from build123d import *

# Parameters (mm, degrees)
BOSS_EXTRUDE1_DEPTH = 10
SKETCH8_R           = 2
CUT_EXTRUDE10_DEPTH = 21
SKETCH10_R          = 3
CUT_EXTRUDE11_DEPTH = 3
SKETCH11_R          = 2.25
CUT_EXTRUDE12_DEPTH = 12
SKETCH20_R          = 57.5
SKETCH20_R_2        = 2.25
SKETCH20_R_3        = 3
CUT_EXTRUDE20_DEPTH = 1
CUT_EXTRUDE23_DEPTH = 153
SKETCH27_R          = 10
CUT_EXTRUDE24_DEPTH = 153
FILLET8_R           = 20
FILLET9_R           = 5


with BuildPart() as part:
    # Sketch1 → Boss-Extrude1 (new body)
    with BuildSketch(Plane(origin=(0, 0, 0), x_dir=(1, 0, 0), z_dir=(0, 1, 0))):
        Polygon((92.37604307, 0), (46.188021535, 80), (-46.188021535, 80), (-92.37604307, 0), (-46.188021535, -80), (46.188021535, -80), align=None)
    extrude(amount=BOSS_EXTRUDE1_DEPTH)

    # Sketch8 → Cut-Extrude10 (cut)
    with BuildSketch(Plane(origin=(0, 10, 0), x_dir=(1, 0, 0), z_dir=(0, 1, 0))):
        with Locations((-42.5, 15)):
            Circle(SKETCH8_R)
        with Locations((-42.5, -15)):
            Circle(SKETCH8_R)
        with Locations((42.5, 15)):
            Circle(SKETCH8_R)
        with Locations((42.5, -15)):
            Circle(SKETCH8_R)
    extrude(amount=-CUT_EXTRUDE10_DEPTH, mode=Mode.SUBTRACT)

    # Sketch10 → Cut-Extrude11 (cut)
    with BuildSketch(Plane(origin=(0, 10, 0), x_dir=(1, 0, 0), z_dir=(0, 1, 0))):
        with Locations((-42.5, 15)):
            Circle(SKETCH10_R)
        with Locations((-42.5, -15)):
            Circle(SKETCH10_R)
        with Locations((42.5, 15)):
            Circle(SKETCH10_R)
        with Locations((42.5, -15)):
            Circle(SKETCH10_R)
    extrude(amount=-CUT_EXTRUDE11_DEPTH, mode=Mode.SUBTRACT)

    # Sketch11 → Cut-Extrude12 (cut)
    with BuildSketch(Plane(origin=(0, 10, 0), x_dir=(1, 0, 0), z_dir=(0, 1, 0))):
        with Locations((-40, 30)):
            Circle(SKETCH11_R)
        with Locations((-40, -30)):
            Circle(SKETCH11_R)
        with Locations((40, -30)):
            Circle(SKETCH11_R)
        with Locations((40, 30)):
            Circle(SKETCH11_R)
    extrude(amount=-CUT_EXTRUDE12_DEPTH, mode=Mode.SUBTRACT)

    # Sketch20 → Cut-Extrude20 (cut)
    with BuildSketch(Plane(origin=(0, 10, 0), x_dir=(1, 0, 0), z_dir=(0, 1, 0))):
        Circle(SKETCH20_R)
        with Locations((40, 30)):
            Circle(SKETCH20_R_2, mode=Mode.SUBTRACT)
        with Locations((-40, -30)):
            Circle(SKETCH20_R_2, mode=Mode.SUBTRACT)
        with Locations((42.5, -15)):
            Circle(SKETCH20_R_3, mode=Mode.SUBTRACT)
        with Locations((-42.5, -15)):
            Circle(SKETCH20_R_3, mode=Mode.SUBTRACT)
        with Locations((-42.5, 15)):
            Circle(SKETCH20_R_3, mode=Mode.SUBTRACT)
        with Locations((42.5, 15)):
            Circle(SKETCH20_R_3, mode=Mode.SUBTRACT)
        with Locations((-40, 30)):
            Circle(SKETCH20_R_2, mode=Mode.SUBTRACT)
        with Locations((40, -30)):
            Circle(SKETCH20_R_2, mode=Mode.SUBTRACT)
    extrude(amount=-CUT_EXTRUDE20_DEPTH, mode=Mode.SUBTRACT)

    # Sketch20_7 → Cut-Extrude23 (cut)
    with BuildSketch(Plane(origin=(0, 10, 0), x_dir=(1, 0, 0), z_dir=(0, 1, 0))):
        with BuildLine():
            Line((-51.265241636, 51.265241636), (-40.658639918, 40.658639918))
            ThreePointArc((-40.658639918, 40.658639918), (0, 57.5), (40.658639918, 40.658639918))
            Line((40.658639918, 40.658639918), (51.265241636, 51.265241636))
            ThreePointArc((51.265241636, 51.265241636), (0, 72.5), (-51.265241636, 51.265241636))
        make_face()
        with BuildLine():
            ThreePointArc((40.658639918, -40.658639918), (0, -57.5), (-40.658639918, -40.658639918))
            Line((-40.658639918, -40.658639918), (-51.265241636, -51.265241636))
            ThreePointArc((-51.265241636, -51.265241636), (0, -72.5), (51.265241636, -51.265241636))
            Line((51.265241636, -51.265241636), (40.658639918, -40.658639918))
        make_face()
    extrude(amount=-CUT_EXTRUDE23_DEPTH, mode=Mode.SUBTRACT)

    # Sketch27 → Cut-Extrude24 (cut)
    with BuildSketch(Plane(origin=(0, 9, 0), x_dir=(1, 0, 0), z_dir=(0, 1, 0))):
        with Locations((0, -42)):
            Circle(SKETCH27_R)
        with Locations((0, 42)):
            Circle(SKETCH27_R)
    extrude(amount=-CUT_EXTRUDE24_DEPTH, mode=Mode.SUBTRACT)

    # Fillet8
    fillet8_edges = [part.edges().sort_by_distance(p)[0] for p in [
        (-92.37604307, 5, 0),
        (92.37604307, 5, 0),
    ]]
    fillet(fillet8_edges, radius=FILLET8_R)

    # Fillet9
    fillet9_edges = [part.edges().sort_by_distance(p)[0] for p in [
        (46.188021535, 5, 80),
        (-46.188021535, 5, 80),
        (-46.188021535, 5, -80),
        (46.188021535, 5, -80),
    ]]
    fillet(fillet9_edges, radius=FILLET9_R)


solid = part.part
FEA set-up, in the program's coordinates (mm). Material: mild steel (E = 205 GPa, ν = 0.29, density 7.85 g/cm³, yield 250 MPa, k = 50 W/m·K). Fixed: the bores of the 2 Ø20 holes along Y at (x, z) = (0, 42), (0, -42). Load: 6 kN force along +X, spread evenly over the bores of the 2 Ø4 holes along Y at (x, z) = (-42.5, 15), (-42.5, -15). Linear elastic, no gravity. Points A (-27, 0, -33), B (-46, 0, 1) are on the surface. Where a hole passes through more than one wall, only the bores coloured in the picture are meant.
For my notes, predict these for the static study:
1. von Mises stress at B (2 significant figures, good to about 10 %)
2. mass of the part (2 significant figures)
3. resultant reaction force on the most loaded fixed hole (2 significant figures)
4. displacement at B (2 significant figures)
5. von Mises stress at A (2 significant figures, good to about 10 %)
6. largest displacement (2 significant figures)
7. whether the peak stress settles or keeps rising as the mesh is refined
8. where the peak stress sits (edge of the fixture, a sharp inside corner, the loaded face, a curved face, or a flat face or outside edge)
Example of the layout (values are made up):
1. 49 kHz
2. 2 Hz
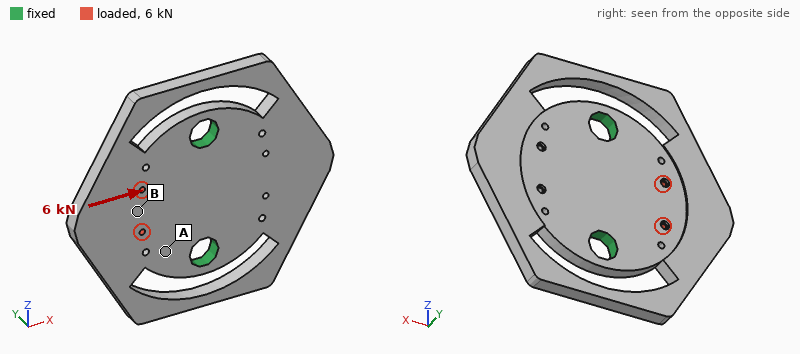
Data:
1. 4.1 MPa
2. 1.4 kg
3. 3.1 kN
4. 4.6 µm
5. 11 MPa
6. 11 µm
7. keeps rising
8. a sharp inside corner
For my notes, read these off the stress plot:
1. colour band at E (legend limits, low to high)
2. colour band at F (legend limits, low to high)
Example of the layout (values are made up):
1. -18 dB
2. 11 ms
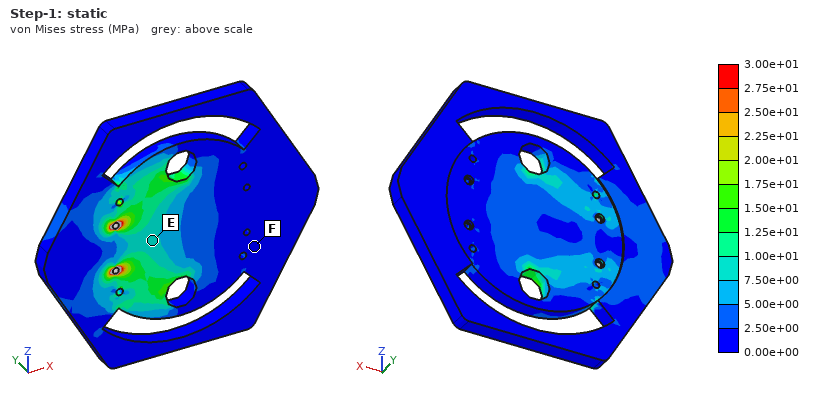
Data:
1. 7.50e+00 to 1.00e+01 MPa
2. 0.00e+00 to 2.50e+00 MPa
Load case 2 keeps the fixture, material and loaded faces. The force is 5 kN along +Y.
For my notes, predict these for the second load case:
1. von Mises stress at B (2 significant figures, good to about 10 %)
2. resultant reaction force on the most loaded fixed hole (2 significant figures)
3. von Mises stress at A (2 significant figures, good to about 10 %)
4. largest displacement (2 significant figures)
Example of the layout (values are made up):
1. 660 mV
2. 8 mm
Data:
1. 22 MPa
2. 2.5 kN
3. 58 MPa
4. 0.21 mm
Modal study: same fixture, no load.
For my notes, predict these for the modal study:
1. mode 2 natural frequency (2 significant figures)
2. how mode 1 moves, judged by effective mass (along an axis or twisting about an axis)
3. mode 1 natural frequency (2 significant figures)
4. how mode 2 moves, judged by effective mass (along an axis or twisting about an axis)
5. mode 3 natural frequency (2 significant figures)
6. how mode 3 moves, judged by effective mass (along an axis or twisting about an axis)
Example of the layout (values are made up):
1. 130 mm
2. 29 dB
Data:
1. 1300 Hz
2. twisting about Z
3. 1200 Hz
4. along Y
5. 1400 Hz
6. twisting about X
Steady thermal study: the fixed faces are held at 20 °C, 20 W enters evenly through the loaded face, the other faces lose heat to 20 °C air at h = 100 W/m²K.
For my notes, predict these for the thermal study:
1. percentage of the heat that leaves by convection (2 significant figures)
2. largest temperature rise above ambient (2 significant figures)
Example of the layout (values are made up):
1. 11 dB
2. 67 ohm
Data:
1. 62 %
2. 17 K
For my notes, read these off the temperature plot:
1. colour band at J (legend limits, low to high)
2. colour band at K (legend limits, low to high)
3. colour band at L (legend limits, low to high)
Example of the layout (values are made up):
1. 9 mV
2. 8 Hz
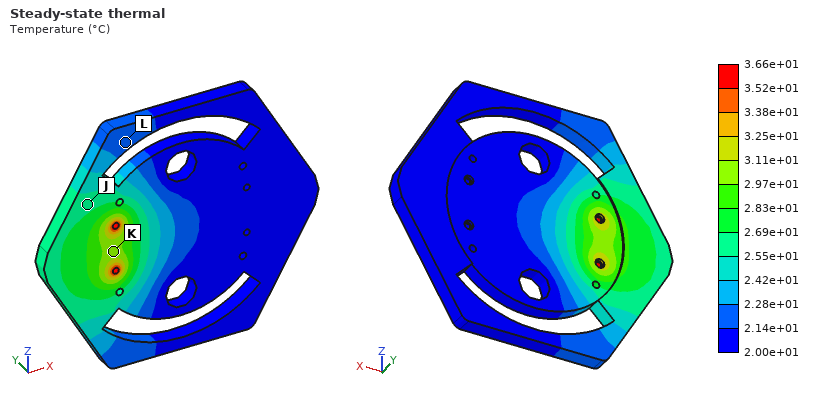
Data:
1. 2.55e+01 to 2.69e+01 °C
2. 2.97e+01 to 3.11e+01 °C
3. 2.14e+01 to 2.28e+01 °C
